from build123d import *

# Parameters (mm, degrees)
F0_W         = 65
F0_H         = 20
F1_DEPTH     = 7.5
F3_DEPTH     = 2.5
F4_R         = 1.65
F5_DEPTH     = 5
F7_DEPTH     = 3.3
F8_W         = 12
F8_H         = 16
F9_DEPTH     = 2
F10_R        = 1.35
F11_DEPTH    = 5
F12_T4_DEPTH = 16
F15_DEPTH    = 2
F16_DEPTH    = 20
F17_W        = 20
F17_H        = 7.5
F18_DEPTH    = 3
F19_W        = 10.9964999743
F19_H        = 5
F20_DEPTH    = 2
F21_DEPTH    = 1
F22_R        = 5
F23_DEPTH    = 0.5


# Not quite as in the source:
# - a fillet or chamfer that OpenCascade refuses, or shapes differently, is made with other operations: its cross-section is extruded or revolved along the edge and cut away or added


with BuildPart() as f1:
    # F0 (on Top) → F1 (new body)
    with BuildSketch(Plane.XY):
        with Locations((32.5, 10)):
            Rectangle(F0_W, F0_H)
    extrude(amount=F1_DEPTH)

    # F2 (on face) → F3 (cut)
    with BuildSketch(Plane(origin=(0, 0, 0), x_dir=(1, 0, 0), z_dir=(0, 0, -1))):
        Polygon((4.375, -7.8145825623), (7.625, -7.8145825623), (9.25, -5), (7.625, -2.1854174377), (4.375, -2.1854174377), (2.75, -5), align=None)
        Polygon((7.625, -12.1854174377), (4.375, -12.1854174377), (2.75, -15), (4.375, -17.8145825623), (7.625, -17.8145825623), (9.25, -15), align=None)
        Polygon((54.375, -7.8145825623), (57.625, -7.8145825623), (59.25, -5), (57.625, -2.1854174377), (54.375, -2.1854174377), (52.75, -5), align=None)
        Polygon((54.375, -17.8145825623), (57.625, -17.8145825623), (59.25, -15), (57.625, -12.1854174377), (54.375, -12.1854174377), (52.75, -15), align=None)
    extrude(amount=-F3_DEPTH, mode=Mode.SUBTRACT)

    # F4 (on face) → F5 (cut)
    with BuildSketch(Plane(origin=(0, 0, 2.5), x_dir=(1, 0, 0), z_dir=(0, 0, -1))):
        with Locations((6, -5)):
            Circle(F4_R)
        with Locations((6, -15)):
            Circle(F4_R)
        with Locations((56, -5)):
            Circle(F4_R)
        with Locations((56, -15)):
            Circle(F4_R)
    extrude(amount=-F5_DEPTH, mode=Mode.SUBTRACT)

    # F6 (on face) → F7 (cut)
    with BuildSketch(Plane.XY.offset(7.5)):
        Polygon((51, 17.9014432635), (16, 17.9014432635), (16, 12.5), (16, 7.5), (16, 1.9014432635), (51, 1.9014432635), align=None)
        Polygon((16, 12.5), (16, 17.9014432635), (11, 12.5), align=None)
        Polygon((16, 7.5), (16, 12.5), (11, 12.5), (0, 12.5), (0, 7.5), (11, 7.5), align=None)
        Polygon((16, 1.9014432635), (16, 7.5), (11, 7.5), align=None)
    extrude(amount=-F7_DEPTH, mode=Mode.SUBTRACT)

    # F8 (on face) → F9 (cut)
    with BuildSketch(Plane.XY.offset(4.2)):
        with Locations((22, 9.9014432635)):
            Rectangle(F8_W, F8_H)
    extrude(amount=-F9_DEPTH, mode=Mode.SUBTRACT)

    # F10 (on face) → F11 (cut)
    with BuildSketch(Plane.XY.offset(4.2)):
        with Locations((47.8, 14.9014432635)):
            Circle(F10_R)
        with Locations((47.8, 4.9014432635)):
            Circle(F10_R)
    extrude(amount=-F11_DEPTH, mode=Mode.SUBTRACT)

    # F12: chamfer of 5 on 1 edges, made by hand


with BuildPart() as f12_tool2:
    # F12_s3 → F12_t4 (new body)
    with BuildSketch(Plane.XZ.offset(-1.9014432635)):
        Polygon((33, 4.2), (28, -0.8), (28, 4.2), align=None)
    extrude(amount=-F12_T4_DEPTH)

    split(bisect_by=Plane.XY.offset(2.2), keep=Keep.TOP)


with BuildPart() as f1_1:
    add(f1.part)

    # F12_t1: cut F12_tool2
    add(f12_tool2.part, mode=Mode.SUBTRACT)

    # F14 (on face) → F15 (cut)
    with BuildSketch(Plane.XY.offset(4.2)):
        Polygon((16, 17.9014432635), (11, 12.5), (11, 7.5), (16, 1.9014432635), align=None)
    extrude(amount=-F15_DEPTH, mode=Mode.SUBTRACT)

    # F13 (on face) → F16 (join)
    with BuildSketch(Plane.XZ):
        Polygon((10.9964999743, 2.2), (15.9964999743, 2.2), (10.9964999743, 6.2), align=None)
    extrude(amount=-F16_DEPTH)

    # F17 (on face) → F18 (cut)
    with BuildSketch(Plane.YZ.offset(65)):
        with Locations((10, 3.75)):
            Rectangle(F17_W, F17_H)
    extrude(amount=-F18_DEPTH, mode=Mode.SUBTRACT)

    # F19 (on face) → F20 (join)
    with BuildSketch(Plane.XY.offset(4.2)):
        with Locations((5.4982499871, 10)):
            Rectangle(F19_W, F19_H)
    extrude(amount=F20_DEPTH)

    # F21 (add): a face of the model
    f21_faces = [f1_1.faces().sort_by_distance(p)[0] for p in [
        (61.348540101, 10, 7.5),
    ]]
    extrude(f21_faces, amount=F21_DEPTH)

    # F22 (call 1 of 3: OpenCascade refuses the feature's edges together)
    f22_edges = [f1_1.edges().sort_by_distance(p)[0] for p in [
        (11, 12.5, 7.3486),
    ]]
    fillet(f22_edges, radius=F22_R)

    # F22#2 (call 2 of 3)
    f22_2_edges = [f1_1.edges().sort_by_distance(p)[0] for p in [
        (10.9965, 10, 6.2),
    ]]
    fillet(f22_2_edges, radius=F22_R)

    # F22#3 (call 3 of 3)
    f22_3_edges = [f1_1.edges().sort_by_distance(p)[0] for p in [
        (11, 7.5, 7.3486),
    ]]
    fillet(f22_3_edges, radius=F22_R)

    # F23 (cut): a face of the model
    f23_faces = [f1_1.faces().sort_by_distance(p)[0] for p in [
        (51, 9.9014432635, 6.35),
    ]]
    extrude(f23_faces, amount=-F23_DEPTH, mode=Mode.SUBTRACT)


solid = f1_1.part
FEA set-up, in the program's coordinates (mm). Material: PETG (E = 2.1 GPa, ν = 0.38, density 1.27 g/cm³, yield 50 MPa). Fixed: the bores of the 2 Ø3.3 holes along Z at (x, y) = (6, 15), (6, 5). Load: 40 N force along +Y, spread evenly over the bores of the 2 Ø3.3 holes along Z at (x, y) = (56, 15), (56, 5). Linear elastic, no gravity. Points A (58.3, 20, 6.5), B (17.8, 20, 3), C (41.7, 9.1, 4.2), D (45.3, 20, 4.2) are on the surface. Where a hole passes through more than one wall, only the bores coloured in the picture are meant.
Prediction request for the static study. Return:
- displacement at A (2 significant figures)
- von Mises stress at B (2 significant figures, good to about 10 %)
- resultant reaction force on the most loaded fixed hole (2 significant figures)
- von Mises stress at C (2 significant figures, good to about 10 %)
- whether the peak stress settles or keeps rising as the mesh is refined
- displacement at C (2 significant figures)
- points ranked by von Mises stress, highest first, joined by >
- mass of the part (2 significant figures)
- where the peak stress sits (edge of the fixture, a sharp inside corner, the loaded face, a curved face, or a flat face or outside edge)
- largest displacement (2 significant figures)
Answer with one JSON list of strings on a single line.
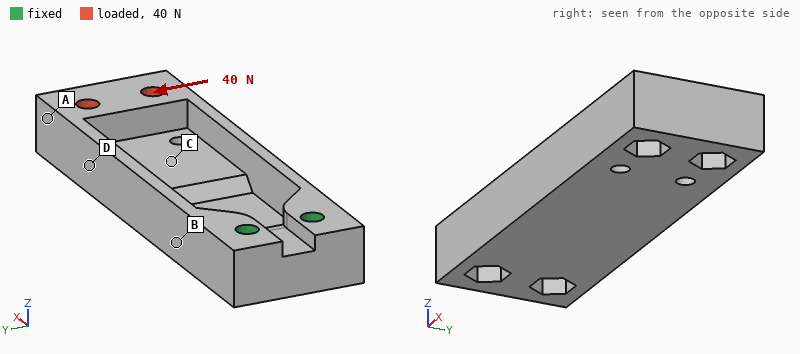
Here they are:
["0.58 mm", "6.3 MPa", "150 N", "3.9 MPa", "keeps rising", "0.30 mm", "B > C > D > A", "8.5 g", "edge of the fixture", "0.66 mm"]
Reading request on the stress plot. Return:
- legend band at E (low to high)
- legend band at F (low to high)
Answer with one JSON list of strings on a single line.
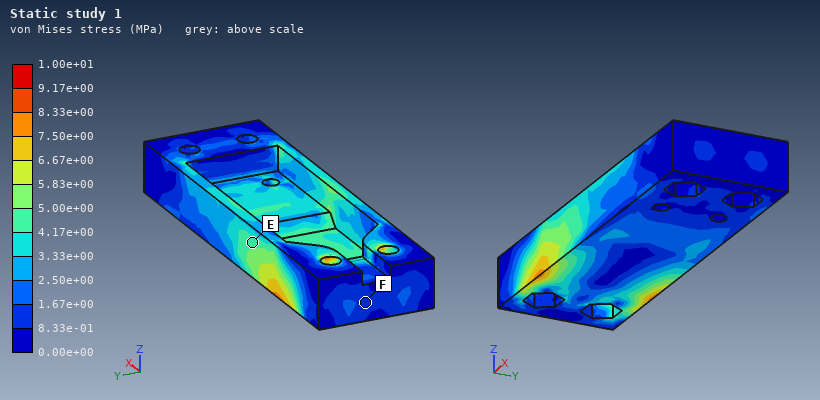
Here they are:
["4.17e+00 to 5.00e+00 MPa", "8.33e-01 to 1.67e+00 MPa"]
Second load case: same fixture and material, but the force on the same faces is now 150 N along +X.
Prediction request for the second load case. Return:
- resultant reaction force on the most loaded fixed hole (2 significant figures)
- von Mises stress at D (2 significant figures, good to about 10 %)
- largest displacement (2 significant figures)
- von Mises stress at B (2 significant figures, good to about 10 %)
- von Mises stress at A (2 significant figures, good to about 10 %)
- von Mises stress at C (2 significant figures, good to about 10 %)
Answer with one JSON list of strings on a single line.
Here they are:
["75 N", "2.7 MPa", "0.69 mm", "1.6 MPa", "0.87 MPa", "2.6 MPa"]
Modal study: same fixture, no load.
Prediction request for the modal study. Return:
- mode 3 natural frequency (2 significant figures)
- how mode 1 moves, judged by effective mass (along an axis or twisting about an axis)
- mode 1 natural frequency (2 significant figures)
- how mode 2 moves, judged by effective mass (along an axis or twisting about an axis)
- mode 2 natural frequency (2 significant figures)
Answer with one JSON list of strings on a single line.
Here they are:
["1500 Hz", "along Z", "410 Hz", "along Y", "800 Hz"]
